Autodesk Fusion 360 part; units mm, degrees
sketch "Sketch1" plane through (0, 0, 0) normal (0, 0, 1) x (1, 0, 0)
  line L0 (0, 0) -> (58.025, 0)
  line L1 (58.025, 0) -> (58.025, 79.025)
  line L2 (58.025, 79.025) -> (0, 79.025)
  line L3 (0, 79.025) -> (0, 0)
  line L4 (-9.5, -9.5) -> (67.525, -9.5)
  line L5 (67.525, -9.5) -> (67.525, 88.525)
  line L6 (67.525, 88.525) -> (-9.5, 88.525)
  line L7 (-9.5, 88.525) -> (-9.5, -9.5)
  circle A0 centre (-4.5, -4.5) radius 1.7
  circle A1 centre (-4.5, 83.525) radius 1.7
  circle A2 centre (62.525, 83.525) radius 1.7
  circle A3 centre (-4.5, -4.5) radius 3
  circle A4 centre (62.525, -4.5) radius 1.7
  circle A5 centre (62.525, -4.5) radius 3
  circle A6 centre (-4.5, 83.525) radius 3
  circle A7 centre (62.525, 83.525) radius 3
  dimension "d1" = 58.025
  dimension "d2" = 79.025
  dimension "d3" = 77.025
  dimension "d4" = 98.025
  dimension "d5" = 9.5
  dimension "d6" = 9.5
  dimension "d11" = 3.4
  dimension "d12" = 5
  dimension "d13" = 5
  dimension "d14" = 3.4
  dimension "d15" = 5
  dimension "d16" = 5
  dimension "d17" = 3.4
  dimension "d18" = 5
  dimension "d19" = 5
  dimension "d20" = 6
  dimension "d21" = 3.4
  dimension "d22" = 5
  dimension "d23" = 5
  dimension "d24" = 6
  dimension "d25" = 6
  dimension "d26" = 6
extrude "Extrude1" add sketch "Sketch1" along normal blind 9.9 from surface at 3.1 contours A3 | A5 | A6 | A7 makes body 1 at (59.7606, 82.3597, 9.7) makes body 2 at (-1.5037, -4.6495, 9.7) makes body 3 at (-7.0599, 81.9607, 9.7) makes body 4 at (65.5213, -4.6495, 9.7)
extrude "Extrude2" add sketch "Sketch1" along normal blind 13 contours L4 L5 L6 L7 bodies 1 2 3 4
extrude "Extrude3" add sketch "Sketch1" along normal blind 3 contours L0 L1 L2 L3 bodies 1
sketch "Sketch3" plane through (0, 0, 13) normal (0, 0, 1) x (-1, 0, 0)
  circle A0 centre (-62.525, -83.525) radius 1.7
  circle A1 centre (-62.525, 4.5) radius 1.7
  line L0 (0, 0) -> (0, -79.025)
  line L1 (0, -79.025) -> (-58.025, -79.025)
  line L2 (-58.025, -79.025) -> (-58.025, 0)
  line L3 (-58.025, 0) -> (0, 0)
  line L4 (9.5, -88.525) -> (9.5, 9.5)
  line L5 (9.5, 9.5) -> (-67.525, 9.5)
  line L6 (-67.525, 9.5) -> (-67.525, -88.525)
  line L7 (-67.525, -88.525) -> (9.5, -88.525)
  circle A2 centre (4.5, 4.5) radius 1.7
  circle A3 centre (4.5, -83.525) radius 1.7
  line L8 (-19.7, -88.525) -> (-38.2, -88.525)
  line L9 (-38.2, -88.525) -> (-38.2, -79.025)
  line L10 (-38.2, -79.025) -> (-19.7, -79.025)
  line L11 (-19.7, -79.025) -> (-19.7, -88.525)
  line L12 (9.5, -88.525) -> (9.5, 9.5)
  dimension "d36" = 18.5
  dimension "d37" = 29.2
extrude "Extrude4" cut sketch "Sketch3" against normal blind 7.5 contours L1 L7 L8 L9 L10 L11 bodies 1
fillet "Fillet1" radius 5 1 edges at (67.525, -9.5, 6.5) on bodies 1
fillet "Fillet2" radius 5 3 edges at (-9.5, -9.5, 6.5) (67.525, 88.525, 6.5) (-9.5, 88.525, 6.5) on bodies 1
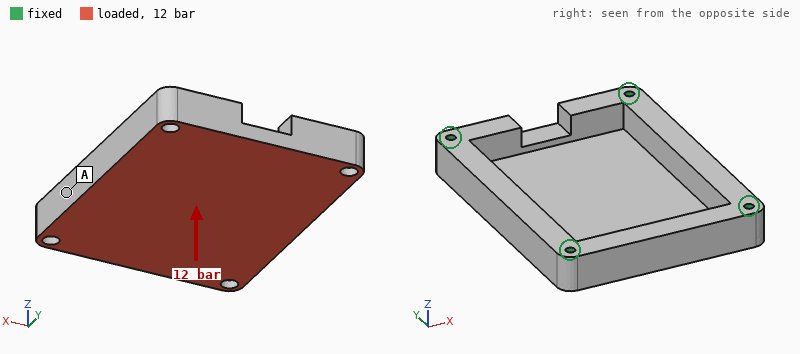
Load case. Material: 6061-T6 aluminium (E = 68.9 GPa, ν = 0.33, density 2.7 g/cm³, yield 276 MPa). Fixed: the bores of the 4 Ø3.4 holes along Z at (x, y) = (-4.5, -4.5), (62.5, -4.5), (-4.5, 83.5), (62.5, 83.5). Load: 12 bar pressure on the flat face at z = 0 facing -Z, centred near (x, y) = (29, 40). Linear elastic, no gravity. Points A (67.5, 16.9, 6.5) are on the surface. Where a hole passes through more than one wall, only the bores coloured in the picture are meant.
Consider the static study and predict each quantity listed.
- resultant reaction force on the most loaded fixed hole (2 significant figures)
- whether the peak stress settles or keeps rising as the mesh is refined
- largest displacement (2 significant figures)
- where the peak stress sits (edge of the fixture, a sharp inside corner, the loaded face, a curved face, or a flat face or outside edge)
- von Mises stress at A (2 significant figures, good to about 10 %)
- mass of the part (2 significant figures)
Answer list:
3.3 kN
keeps rising
0.31 mm
edge of the fixture
18 MPa
130 g
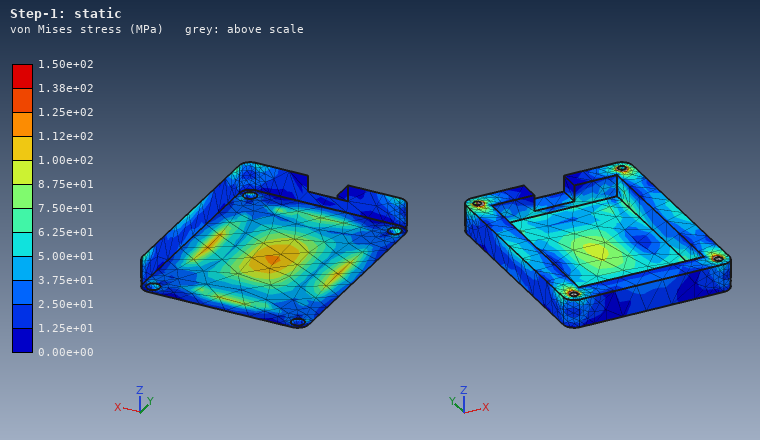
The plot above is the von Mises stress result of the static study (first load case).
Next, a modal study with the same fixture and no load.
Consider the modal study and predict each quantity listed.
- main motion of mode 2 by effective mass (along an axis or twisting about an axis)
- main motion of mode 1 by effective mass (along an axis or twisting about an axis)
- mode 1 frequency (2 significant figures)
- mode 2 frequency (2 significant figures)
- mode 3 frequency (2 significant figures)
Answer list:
twisting about Y
along Z
4300 Hz
6400 Hz
7700 Hz
